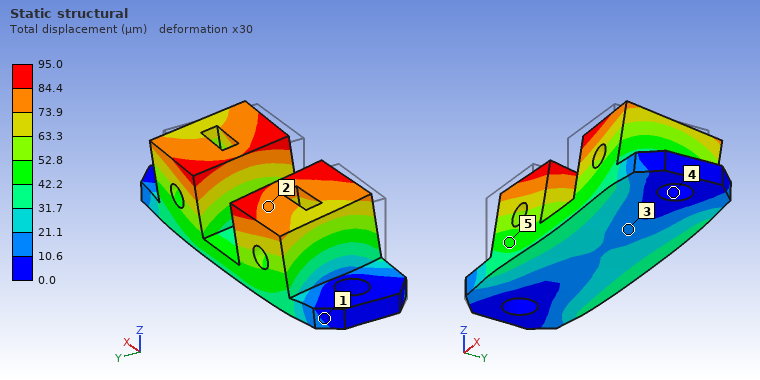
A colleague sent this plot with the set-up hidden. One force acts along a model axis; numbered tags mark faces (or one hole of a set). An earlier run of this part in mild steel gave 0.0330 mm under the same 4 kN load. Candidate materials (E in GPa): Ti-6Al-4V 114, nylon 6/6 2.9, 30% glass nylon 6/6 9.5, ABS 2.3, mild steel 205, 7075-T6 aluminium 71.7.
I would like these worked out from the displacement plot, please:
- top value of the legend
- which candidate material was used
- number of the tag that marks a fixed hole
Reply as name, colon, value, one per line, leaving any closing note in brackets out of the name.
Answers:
top value of the legend: 95.0 µm
which candidate material was used: 7075-T6 aluminium
number of the tag that marks a fixed hole: 4
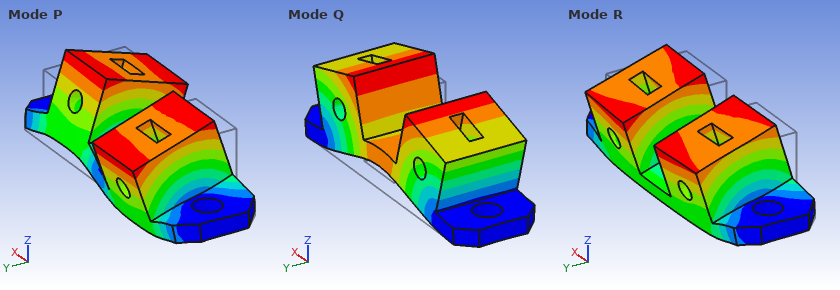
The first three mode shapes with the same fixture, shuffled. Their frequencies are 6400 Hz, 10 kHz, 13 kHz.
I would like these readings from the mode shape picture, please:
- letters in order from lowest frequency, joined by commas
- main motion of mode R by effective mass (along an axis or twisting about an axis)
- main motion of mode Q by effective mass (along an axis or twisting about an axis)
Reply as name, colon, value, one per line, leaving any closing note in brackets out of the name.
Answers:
letters in order from lowest frequency, joined by commas: Q, R, P
main motion of mode R by effective mass: along Y
main motion of mode Q by effective mass: along Z
